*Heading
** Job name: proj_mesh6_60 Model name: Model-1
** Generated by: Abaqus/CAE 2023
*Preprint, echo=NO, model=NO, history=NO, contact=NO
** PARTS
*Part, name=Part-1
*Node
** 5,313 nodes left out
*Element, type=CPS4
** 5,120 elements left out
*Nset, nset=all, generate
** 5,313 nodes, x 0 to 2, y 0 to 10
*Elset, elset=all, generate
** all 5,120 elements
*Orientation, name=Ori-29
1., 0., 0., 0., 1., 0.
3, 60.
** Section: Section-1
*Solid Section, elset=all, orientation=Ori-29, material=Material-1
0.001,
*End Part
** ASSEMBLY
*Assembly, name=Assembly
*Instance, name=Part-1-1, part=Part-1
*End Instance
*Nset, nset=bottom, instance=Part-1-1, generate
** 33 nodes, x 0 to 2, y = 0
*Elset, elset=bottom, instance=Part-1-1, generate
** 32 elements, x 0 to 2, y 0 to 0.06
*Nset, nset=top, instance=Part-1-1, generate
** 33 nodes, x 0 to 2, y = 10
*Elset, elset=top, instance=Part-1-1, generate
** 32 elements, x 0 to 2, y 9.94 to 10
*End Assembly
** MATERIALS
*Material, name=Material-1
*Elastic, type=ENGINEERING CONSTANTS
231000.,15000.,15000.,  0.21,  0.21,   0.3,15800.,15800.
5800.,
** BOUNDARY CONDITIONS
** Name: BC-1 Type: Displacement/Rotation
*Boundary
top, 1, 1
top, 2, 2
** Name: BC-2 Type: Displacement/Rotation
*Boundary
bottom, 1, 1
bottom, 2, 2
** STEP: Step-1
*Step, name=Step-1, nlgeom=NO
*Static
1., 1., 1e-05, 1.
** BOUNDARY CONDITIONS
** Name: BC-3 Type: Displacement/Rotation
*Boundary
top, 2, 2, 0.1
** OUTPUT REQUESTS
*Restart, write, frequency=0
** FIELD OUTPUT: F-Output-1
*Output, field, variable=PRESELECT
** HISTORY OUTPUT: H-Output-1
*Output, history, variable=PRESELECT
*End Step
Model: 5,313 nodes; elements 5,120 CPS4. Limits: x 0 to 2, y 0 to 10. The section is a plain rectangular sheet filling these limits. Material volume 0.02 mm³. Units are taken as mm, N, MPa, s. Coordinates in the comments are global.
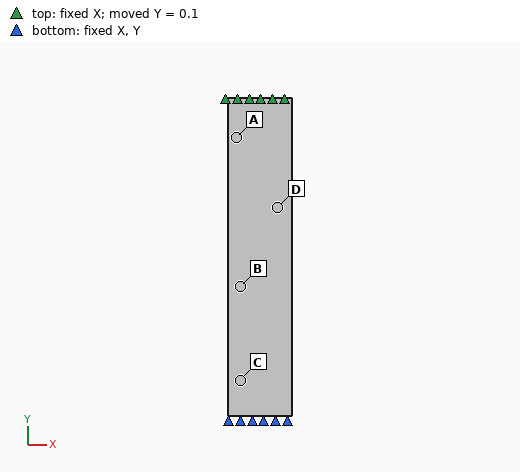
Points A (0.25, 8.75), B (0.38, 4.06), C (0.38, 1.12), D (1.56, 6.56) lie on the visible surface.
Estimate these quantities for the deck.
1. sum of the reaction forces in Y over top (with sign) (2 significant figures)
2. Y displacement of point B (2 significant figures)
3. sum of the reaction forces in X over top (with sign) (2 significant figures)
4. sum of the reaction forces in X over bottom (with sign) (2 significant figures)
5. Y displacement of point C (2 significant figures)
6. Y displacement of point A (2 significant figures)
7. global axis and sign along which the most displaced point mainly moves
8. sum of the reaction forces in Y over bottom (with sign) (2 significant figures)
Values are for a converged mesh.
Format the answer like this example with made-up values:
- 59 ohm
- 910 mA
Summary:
- 1.2 N
- 0.053 mm
- 0.065 N
- -0.065 N
- 0.016 mm
- 0.092 mm
- +Y
- -1.2 N
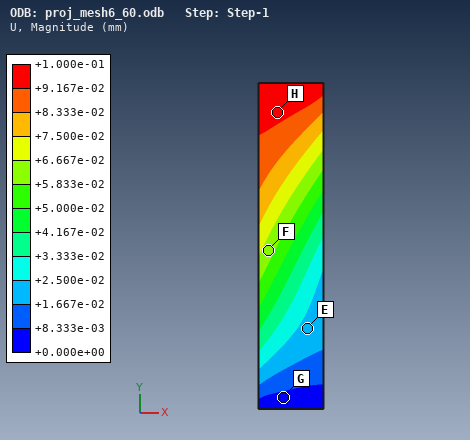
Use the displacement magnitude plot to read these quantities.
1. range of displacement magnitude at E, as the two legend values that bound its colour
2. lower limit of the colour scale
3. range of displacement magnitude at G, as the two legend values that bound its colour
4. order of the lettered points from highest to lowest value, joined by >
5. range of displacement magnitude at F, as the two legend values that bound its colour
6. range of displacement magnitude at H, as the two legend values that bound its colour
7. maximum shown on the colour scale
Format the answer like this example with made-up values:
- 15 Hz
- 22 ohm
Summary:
- +1.667e-02 to +2.500e-02 mm
- +0.000e+00 mm
- +0.000e+00 to +8.333e-03 mm
- H > F > E > G
- +5.833e-02 to +6.667e-02 mm
- +9.167e-02 to +1.000e-01 mm
- +1.000e-01 mm
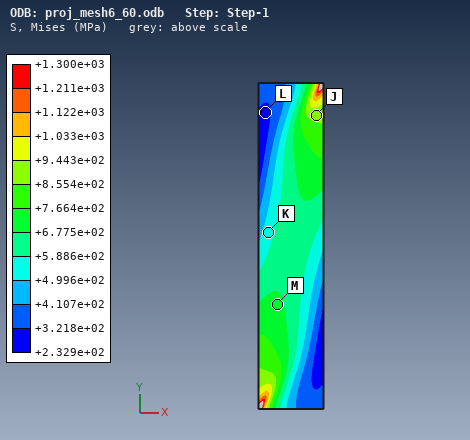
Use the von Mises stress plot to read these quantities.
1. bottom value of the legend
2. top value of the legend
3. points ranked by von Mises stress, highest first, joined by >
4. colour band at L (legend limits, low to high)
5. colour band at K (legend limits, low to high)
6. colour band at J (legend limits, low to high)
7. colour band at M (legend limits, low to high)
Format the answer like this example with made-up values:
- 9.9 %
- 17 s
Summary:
- +2.329e+02 MPa
- +1.300e+03 MPa
- J > M > K > L
- +2.329e+02 to +3.218e+02 MPa
- +4.996e+02 to +5.886e+02 MPa
- +8.554e+02 to +9.443e+02 MPa
- +6.775e+02 to +7.664e+02 MPa
